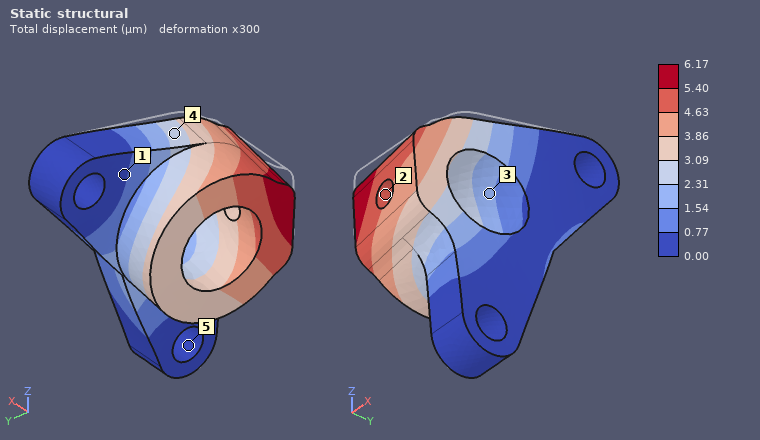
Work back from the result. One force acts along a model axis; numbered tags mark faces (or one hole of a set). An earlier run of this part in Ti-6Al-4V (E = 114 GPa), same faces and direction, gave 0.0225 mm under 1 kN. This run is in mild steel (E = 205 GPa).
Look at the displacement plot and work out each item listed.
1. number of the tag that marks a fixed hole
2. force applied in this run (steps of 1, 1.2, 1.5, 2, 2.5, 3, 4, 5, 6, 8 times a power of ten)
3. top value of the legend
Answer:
5
500 N
6.17 µm
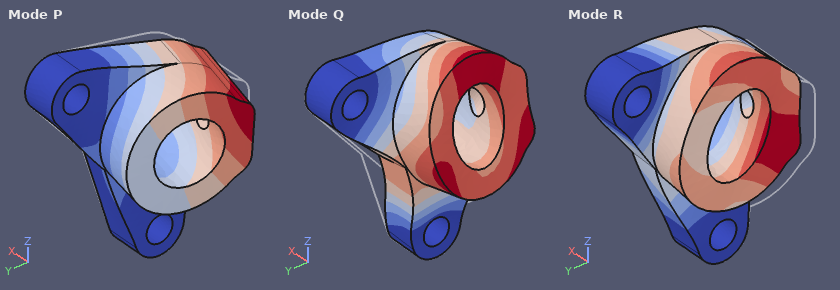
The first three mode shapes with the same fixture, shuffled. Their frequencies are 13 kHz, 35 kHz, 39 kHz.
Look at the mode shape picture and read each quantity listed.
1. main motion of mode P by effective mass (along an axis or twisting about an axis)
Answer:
along X
